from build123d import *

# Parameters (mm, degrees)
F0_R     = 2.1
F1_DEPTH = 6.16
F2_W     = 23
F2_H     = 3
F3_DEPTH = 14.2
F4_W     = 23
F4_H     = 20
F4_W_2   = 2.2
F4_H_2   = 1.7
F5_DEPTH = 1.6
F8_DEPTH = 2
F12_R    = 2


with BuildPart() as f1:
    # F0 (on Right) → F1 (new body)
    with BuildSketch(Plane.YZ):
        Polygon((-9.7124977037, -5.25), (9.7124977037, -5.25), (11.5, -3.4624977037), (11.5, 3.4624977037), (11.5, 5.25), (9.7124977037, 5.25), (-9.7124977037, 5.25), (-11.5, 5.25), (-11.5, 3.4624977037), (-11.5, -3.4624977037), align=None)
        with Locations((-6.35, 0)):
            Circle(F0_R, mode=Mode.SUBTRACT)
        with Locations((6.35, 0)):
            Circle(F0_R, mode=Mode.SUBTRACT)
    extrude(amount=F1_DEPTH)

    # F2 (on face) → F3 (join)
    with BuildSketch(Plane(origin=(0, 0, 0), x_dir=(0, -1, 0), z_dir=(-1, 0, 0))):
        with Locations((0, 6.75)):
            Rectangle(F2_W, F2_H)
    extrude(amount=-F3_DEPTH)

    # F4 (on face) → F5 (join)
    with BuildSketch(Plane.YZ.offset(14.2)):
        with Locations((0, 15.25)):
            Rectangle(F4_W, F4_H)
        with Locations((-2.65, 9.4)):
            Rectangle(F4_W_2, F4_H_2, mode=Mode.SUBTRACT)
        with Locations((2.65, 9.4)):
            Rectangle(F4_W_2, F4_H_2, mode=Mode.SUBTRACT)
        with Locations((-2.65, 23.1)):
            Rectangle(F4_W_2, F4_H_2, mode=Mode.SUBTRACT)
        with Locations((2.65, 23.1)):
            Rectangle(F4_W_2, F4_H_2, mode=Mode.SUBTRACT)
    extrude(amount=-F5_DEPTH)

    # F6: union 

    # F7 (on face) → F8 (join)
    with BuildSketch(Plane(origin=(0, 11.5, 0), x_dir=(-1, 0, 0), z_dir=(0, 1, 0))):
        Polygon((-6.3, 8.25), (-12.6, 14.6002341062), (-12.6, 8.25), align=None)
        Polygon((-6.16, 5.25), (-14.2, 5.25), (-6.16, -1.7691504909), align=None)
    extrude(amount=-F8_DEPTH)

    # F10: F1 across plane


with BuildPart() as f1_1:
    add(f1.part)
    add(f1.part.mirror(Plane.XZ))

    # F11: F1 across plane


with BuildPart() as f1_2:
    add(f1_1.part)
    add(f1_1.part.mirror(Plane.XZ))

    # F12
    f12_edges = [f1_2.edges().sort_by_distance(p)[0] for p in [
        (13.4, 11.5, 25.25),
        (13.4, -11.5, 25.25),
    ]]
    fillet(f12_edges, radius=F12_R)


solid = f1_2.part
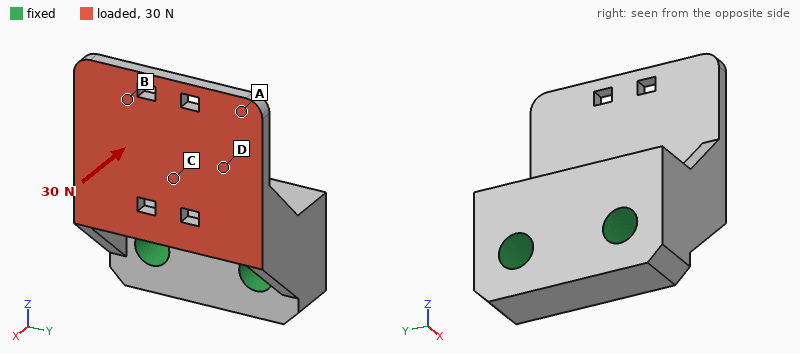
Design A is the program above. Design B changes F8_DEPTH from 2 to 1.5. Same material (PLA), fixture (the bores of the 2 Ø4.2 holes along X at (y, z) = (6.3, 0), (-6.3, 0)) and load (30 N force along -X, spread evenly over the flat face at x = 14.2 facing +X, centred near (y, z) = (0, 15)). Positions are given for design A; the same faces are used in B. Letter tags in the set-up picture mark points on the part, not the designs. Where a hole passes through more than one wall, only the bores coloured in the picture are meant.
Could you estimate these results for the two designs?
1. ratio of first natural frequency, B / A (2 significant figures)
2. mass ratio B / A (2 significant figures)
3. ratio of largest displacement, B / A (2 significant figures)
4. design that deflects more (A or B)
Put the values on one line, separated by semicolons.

0.94; 0.98; 1.1; B
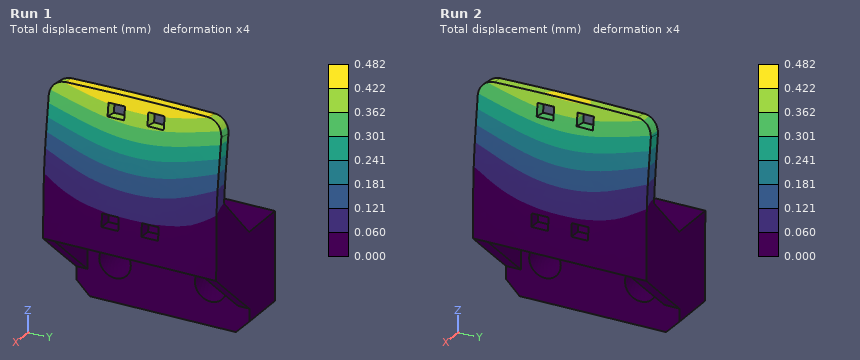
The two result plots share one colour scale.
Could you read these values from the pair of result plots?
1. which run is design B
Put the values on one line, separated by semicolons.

Run 1
